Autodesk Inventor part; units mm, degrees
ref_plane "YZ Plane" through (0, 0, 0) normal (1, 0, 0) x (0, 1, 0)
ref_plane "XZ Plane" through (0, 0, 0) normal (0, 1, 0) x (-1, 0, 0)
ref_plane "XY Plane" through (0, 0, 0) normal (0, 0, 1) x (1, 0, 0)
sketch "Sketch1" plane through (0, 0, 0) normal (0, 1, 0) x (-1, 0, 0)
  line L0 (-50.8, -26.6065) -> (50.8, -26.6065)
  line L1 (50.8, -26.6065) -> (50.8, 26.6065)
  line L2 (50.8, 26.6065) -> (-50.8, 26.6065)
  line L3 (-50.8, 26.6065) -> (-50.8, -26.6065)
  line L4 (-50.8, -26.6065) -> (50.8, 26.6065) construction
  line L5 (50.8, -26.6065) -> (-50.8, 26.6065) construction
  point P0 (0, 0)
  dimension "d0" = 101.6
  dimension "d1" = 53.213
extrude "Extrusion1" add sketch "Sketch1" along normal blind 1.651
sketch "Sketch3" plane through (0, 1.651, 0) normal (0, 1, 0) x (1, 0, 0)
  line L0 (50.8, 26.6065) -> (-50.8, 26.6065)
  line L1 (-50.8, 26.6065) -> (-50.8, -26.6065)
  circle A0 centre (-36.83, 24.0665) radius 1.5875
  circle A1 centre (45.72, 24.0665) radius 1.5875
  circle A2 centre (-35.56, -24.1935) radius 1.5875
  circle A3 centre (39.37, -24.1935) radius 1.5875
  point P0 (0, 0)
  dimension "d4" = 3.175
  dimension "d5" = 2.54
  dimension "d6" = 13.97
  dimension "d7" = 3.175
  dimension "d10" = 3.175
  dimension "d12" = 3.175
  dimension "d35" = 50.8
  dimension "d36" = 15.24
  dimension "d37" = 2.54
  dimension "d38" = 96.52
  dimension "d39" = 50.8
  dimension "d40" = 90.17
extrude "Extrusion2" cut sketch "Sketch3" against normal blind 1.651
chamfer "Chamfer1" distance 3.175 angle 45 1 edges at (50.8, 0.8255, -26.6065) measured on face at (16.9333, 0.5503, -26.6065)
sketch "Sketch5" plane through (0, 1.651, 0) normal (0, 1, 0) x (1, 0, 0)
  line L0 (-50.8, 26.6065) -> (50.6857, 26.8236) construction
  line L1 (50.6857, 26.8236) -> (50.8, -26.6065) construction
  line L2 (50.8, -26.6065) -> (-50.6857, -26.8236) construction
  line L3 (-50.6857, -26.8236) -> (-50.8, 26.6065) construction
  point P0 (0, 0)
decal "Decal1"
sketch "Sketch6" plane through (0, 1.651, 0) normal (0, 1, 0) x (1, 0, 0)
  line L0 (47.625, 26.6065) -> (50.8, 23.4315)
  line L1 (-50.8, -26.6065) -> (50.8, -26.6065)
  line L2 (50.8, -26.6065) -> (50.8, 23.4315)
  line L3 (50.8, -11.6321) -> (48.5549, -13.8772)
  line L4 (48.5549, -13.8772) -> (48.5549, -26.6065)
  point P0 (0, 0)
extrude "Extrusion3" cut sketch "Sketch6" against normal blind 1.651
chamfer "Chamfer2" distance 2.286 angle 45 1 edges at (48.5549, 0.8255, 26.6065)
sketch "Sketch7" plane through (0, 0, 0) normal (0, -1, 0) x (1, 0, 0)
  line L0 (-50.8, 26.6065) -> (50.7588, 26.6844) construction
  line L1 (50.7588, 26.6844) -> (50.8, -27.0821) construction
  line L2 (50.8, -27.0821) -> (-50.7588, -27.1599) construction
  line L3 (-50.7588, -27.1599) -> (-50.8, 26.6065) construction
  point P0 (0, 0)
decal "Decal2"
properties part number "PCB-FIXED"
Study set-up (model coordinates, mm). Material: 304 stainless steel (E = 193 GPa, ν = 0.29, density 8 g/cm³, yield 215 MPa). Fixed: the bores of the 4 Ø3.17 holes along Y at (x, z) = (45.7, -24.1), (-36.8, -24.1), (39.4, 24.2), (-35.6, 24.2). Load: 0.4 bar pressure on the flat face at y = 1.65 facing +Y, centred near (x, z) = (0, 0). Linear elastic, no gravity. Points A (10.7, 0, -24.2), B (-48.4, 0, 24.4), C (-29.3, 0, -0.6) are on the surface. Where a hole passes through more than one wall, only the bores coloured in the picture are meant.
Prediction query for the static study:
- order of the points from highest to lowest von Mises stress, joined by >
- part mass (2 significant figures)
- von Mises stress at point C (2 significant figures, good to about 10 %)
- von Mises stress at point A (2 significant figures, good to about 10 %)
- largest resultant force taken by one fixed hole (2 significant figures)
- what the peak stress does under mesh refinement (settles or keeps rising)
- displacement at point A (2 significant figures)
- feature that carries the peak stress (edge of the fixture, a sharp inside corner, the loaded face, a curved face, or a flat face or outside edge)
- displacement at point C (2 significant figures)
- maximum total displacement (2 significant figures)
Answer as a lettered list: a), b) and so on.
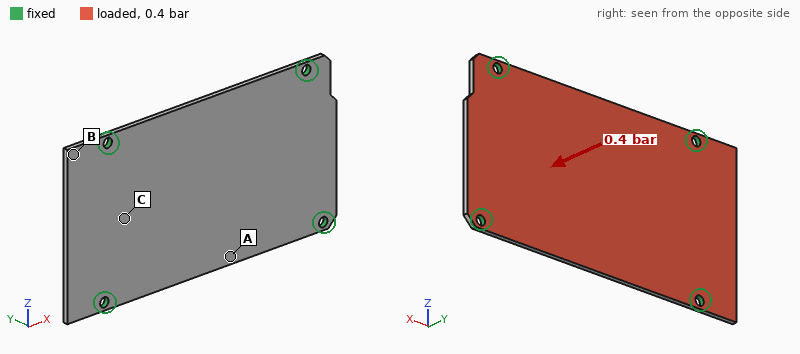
a) A > C > B
b) 70 g
c) 17 MPa
d) 28 MPa
e) 59 N
f) keeps rising
g) 81 µm
h) edge of the fixture
i) 27 µm
j) 86 µm
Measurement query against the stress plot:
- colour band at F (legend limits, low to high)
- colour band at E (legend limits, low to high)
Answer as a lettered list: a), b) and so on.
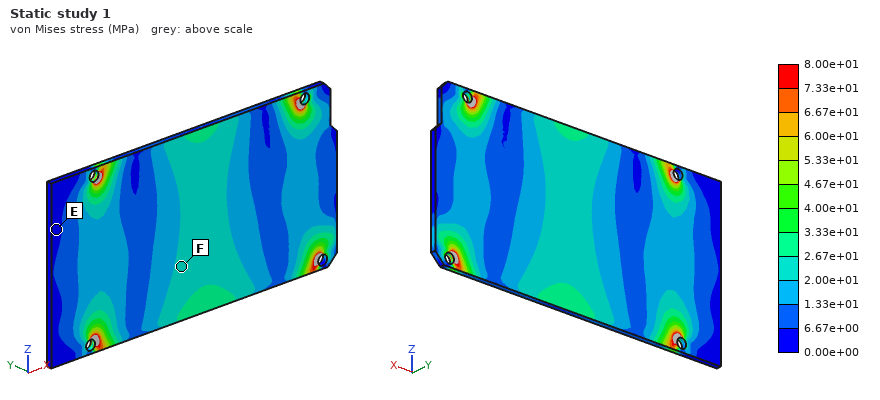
a) 2.00e+01 to 2.67e+01 MPa
b) 0.00e+00 to 6.67e+00 MPa
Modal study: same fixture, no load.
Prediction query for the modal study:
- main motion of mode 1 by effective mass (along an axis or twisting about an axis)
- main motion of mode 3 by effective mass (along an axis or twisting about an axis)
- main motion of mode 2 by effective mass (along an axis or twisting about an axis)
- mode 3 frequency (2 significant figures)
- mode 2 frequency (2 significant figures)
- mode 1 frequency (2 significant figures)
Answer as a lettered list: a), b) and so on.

a) along Y
b) twisting about Z
c) twisting about X
d) 2900 Hz
e) 1900 Hz
f) 1100 Hz
